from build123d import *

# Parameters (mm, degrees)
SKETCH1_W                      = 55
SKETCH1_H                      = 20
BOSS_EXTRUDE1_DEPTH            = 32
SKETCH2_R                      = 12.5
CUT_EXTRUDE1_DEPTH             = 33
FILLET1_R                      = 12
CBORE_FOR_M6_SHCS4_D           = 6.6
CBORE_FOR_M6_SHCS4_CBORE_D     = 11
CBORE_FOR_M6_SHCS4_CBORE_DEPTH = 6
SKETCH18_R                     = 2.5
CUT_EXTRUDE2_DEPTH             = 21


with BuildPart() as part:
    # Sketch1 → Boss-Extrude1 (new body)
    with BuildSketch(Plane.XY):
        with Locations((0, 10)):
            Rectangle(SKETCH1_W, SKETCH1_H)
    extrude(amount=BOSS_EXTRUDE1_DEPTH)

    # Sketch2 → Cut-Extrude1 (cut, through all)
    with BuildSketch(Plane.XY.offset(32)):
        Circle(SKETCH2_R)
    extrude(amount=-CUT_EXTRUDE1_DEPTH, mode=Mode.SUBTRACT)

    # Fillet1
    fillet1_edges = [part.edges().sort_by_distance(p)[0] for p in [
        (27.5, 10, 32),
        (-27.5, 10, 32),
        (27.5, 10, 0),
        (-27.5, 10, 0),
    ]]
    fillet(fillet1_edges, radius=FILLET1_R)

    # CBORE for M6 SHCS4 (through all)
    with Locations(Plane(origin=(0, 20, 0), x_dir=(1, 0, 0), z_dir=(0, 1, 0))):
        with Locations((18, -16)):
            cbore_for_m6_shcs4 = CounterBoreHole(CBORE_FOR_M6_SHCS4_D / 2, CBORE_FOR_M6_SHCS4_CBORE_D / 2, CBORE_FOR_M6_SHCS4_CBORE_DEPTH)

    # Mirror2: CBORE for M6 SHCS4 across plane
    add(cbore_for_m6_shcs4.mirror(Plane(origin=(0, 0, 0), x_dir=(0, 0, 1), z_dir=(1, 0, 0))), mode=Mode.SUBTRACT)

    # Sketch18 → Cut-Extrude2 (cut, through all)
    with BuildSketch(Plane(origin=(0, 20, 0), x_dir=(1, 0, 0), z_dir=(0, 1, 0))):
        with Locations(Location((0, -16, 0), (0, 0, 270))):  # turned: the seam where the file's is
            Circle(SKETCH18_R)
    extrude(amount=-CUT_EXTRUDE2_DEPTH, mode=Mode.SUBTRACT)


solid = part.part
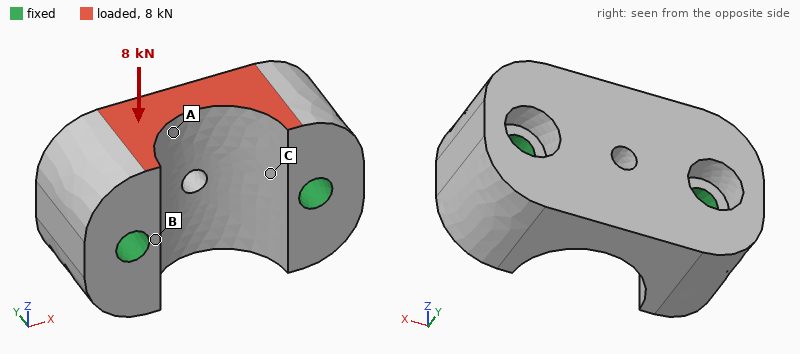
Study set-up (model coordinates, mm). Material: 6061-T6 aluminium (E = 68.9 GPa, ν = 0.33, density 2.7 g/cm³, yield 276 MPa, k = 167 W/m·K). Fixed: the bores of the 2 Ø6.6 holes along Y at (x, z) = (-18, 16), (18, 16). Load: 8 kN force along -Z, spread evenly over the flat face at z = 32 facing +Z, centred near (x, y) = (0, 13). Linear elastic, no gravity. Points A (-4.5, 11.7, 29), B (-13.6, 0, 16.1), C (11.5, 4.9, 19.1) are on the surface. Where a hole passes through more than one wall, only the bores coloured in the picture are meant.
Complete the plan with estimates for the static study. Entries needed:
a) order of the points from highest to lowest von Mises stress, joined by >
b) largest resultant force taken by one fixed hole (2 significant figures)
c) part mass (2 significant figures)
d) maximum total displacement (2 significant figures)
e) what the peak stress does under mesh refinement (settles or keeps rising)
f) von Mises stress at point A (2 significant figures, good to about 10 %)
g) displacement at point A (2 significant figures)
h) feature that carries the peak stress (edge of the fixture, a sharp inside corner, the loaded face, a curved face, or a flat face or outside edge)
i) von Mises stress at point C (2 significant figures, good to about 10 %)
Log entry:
A > C > B
4.0 kN
61 g
19 µm
keeps rising
24 MPa
12 µm
edge of the fixture
14 MPa
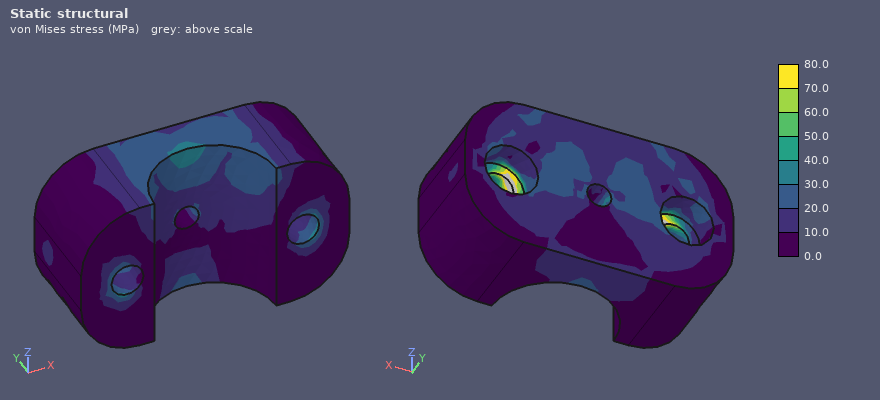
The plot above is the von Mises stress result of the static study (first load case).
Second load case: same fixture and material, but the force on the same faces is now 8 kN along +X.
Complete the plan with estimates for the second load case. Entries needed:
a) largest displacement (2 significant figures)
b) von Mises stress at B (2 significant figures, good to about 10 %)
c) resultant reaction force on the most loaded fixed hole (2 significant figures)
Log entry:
17 µm
22 MPa
4.8 kN
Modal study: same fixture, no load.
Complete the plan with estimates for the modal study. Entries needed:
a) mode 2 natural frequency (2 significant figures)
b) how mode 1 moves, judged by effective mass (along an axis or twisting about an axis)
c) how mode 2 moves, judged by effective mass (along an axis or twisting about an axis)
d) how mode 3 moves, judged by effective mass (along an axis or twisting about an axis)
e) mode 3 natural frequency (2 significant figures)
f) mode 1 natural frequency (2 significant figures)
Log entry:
28 kHz
along Z
twisting about Y
along Y
29 kHz
21 kHz
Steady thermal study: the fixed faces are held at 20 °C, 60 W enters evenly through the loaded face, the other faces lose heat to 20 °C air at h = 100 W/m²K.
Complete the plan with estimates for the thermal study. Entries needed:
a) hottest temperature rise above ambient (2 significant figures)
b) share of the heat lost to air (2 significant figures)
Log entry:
15 K
3.2 %
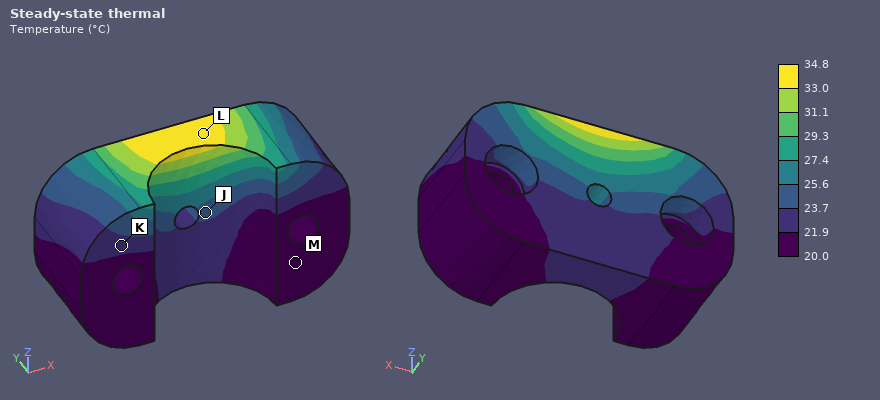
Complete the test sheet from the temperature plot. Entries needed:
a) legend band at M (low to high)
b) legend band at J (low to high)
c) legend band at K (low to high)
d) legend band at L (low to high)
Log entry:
20.0 to 21.9 °C
23.7 to 25.6 °C
21.9 to 23.7 °C
33.0 to 34.8 °C
